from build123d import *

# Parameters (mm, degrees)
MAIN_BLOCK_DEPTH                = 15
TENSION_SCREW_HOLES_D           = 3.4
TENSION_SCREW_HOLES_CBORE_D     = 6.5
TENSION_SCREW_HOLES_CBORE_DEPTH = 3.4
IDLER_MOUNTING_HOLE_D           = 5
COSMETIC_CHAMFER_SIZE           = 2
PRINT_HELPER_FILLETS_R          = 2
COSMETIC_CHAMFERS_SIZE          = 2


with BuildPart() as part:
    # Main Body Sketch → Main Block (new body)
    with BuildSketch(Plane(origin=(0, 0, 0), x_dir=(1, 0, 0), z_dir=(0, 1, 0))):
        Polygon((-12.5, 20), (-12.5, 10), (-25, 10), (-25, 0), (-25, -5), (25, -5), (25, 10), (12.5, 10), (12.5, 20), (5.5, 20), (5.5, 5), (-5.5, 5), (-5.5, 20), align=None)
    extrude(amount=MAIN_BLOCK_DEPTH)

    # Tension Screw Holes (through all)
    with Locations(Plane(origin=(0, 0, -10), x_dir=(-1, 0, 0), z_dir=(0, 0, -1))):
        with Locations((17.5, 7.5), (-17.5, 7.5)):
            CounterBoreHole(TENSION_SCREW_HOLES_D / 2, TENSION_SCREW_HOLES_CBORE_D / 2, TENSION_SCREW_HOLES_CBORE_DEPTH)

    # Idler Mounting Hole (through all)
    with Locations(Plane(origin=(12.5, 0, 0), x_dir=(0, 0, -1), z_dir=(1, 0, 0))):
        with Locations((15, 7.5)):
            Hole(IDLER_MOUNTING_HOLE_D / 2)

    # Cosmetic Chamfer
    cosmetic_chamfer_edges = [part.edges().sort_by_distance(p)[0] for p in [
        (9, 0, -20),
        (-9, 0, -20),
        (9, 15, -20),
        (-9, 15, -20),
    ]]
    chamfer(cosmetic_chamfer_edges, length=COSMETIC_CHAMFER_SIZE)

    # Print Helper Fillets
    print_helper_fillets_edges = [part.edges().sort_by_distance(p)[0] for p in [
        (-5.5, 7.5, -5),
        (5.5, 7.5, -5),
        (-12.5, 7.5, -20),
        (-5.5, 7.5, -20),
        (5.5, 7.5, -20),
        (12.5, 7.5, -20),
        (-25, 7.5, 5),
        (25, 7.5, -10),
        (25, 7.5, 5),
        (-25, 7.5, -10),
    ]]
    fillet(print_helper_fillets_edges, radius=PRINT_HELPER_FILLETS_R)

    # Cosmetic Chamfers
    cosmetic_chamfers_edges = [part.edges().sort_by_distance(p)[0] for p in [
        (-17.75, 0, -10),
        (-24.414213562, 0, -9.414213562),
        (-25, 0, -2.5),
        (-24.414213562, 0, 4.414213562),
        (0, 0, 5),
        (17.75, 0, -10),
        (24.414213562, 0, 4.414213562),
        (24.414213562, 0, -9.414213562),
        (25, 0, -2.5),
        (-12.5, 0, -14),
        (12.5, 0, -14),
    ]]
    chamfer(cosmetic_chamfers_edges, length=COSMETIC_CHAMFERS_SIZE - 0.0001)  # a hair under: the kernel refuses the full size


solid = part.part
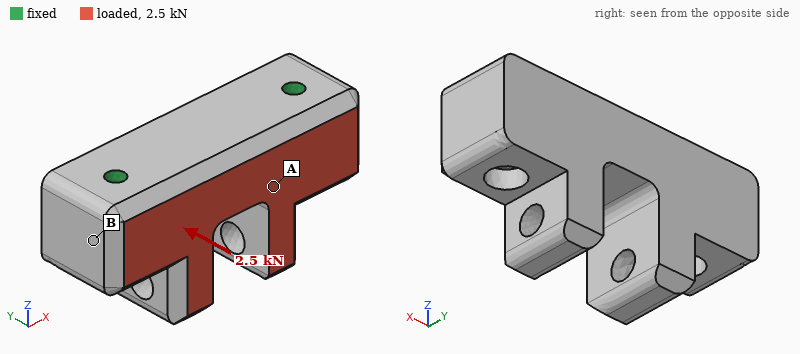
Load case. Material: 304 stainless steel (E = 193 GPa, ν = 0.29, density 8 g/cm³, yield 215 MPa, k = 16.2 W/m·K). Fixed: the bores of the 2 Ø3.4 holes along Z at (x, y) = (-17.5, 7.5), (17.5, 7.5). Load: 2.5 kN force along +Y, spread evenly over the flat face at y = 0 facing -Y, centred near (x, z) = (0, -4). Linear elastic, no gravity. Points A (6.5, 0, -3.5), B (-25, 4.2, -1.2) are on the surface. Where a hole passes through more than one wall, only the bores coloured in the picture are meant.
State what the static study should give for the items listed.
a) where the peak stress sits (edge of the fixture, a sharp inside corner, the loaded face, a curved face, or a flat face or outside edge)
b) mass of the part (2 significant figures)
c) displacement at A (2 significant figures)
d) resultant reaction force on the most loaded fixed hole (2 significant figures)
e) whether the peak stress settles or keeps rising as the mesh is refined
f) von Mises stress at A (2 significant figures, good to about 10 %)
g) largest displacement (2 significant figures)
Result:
edge of the fixture
92 g
1.7 µm
1.3 kN
keeps rising
12 MPa
3.5 µm
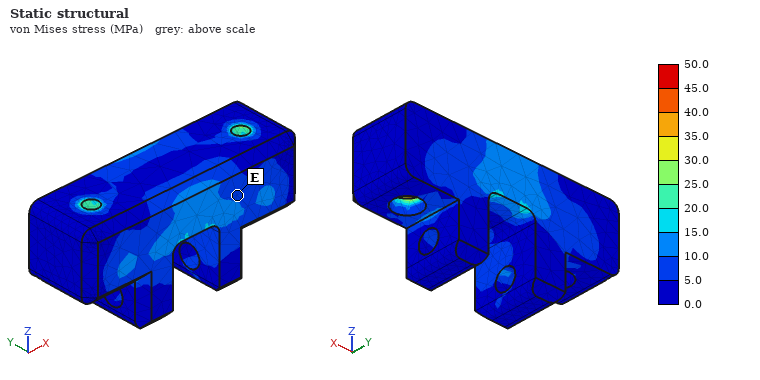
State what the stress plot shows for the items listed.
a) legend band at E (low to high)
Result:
5.0 to 10.0 MPa
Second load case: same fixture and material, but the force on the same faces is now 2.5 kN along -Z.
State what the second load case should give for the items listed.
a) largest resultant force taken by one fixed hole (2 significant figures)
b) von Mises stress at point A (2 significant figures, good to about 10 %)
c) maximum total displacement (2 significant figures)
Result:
1.3 kN
13 MPa
4.8 µm
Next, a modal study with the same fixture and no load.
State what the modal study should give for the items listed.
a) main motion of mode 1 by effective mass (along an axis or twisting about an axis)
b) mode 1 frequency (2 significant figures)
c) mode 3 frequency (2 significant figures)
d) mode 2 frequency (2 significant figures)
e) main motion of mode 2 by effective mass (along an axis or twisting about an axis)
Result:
along Y
18 kHz
23 kHz
19 kHz
along Z
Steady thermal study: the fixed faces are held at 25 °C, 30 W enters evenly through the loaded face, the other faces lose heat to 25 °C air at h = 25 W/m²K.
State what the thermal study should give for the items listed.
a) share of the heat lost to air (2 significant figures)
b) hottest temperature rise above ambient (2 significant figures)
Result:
6.9 %
50 K
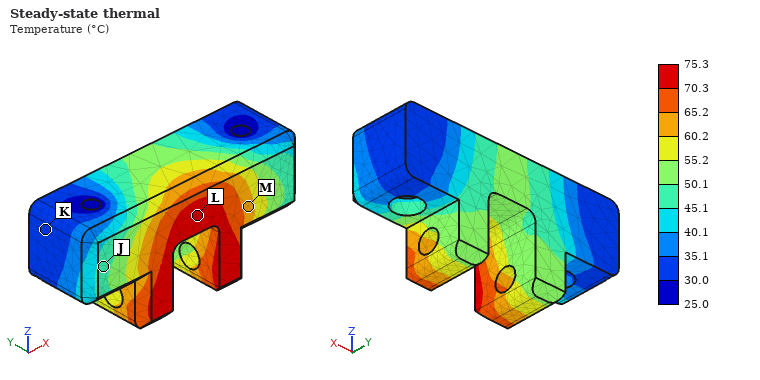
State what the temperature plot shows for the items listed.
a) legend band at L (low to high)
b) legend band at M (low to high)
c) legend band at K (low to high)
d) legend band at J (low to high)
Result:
70.3 to 75.3 °C
60.2 to 65.2 °C
30.0 to 35.1 °C
45.1 to 50.1 °C
